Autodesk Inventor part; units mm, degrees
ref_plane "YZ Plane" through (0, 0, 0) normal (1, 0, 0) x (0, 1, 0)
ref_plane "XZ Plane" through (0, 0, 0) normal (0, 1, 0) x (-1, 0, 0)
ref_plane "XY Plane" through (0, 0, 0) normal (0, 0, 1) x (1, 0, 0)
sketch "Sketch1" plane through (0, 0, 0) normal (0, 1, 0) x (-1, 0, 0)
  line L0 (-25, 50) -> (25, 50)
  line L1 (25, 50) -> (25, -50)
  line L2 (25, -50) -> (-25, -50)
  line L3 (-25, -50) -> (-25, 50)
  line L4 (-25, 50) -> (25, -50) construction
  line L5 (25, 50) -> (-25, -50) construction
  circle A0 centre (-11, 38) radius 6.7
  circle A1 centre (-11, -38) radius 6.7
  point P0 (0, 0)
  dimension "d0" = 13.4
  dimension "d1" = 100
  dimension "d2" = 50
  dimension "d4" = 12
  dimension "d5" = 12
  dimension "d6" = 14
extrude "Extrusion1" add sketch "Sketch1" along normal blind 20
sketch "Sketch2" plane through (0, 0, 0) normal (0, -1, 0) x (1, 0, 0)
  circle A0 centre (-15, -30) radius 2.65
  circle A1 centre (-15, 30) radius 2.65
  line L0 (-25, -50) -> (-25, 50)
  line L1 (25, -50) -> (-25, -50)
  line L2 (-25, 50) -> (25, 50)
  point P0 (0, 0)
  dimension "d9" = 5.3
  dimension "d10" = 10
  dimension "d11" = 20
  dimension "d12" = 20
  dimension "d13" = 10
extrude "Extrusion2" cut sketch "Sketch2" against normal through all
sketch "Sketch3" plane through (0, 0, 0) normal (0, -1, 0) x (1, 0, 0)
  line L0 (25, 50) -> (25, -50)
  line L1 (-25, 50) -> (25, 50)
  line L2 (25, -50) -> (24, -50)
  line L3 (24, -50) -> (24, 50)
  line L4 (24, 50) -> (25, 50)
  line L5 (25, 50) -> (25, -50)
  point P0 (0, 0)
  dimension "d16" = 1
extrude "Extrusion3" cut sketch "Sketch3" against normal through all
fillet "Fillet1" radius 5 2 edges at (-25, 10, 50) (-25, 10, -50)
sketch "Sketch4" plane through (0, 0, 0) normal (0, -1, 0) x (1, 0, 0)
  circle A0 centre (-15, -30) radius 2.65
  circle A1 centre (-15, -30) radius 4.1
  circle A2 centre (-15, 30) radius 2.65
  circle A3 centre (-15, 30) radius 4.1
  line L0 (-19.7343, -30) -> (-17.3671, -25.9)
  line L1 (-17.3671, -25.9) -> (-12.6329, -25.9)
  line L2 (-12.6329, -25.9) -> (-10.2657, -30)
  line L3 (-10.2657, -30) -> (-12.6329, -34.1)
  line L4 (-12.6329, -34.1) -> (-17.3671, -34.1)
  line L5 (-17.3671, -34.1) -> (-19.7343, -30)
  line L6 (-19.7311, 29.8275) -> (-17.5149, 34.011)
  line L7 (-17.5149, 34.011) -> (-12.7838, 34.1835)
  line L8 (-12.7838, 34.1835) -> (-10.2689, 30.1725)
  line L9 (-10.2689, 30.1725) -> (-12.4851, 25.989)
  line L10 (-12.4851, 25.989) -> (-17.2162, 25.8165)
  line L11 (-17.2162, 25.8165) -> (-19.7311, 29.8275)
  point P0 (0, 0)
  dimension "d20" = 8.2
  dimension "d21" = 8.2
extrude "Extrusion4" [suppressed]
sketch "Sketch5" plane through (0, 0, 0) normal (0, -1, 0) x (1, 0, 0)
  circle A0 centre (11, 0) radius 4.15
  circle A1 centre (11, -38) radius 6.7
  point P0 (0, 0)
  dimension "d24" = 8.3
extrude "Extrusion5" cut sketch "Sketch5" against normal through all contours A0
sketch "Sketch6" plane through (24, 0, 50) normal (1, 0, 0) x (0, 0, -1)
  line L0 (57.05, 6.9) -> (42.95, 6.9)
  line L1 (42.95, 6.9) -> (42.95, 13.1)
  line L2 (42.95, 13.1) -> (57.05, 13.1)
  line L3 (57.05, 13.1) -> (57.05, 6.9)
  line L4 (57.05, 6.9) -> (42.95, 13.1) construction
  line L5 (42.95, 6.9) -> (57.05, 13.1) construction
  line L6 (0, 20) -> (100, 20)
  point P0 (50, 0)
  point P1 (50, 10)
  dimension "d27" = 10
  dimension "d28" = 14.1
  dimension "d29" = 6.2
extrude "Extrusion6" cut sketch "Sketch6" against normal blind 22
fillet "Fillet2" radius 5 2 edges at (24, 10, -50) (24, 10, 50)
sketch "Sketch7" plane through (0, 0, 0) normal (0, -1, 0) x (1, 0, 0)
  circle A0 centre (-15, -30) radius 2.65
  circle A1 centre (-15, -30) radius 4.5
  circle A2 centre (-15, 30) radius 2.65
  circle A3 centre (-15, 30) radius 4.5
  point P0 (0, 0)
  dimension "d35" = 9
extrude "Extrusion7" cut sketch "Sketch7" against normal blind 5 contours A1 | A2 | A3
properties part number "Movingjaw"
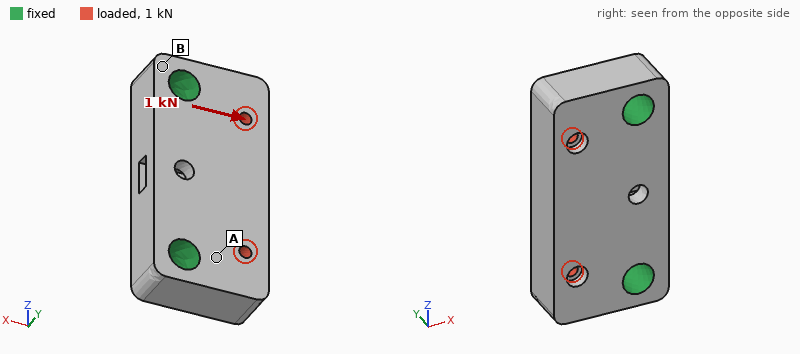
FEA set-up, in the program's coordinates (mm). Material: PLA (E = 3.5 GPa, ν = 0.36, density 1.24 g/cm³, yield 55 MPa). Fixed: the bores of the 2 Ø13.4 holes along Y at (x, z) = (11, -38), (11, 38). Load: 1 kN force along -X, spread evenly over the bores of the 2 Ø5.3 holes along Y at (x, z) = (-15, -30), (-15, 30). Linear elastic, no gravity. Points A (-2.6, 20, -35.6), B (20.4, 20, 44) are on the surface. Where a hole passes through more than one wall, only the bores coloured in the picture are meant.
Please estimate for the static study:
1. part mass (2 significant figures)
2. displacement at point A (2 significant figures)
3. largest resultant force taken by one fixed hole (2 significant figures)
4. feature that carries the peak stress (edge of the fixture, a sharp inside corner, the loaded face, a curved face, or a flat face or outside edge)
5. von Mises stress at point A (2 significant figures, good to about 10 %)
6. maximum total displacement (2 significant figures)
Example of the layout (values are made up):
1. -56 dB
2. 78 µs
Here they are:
1. 110 g
2. 4.7 µm
3. 510 N
4. the loaded face
5. 1.9 MPa
6. 16 µm
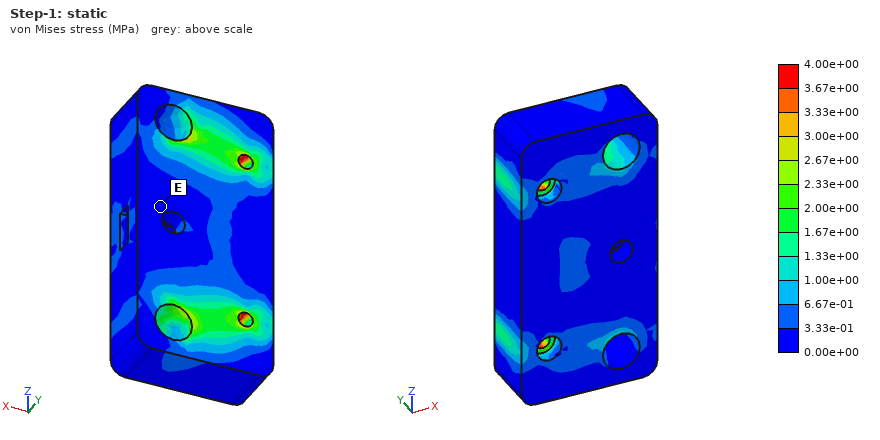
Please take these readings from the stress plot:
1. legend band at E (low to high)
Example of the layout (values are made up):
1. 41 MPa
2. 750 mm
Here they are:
1. 0.00e+00 to 3.33e-01 MPa
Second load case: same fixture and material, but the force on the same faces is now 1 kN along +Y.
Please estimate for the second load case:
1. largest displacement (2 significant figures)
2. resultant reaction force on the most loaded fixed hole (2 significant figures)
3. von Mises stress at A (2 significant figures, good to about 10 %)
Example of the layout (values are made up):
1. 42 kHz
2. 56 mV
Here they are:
1. 69 µm
2. 500 N
3. 3.6 MPa
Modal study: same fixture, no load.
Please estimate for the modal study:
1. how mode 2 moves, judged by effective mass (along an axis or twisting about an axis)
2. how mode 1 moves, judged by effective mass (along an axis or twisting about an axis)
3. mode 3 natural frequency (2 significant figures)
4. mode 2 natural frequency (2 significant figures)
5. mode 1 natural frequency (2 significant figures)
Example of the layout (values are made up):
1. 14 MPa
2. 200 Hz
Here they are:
1. twisting about X
2. along Y
3. 5300 Hz
4. 4700 Hz
5. 2900 Hz
